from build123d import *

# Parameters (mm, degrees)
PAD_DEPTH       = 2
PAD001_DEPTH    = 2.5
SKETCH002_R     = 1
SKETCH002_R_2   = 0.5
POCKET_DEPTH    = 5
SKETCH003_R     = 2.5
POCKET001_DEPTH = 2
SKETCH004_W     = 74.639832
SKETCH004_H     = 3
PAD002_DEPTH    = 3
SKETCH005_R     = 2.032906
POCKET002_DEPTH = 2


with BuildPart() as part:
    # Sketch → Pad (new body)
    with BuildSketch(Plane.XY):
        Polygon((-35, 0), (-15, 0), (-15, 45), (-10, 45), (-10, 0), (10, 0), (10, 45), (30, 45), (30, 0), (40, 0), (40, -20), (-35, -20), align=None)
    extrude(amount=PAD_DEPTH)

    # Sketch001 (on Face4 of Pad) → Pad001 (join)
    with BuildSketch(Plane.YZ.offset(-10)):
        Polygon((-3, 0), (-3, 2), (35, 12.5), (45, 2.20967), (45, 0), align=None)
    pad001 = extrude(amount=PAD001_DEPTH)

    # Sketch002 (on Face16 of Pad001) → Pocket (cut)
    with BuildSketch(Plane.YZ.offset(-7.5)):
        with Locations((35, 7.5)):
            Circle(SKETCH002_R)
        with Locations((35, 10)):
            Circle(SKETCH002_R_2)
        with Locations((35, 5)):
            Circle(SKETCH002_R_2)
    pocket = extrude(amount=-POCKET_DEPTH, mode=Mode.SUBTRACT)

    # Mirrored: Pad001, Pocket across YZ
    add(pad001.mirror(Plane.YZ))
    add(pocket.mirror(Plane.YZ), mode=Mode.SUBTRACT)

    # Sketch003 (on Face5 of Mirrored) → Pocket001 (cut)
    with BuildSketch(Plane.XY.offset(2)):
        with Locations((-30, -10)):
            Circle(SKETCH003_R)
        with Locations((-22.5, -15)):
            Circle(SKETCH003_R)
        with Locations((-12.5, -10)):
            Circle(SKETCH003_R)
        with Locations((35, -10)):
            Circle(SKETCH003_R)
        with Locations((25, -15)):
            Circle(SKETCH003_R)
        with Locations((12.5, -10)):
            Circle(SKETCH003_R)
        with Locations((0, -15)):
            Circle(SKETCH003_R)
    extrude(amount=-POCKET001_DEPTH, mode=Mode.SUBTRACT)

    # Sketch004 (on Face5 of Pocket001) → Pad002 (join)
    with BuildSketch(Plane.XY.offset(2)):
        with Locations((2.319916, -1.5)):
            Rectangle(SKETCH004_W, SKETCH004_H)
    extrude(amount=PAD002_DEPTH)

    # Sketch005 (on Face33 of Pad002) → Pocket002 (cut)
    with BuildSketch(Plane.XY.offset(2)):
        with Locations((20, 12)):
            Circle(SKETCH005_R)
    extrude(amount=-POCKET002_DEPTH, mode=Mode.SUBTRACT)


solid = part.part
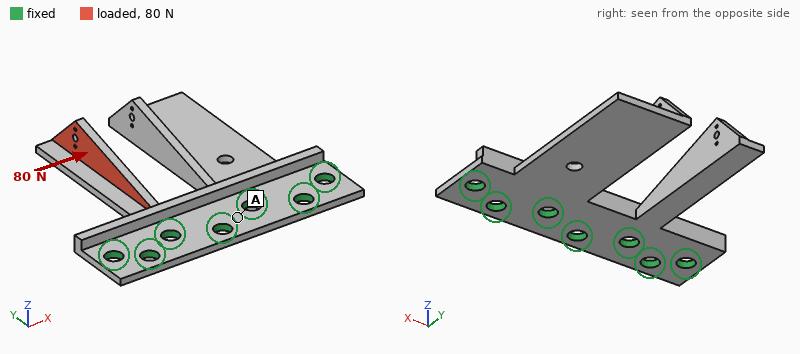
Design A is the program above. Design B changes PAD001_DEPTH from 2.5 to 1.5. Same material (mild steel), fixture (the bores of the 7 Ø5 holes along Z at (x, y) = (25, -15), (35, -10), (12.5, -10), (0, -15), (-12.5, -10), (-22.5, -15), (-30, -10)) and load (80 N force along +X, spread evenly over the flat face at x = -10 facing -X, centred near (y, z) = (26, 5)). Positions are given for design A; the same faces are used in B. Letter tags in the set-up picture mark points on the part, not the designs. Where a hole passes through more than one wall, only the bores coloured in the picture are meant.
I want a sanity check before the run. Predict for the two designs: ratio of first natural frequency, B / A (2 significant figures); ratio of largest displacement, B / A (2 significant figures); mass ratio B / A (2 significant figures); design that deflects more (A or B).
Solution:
1.0
1.7
0.91
B
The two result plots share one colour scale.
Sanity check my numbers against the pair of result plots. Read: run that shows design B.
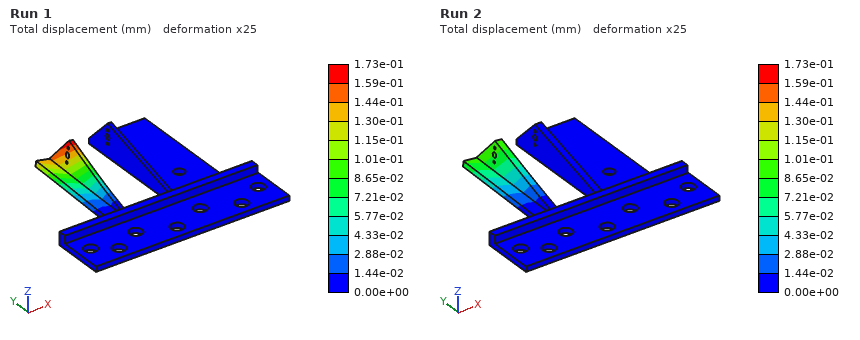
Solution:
Run 1
